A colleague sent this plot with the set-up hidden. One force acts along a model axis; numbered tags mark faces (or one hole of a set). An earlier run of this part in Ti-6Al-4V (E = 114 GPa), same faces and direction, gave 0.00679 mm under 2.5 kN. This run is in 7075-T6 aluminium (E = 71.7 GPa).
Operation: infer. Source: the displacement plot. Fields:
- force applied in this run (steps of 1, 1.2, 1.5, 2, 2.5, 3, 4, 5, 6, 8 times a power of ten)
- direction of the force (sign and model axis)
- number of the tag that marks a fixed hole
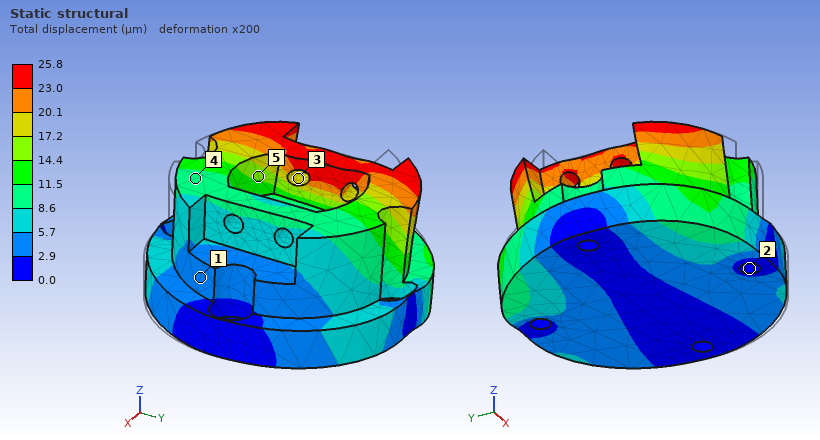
6 kN
+Y
2
